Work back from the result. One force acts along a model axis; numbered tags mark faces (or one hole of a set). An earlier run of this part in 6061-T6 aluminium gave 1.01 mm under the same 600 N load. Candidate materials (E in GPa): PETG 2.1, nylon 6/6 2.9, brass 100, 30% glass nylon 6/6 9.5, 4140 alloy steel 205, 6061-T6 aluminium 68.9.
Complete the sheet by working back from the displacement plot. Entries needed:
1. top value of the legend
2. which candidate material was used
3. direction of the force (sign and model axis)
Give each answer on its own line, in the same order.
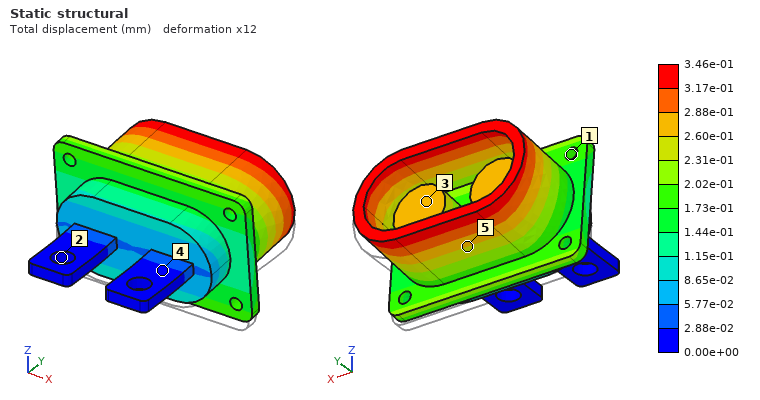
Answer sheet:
3.46e-01 mm
4140 alloy steel
+Z
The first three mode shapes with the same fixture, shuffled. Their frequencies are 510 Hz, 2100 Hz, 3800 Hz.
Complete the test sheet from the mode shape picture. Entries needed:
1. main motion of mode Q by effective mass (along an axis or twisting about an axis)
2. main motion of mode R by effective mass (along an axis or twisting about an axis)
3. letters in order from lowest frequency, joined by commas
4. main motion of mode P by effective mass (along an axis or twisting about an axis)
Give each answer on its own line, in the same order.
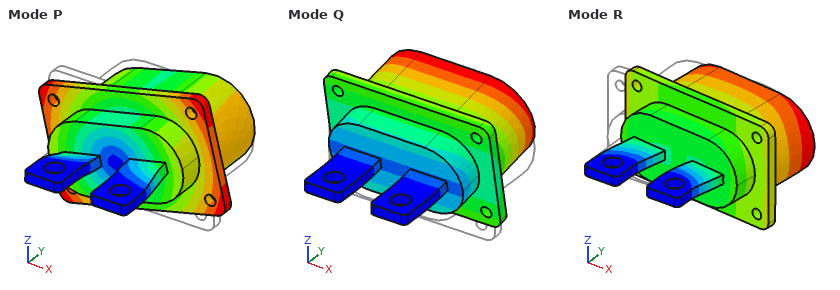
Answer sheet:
along Z
along X
Q, P, R
twisting about Y
